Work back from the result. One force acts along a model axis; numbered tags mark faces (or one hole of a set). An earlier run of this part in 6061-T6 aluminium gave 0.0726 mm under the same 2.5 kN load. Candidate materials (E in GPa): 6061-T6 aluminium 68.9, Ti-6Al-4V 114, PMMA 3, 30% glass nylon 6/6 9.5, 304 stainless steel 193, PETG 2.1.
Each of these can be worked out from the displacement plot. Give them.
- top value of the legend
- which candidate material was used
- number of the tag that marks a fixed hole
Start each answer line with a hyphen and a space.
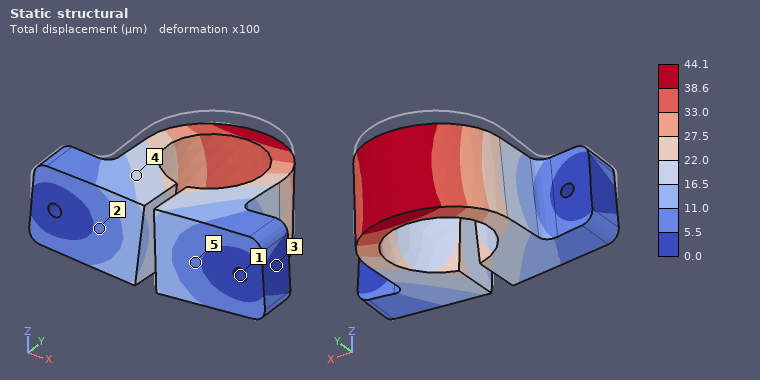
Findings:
- 44.1 µm
- Ti-6Al-4V
- 1
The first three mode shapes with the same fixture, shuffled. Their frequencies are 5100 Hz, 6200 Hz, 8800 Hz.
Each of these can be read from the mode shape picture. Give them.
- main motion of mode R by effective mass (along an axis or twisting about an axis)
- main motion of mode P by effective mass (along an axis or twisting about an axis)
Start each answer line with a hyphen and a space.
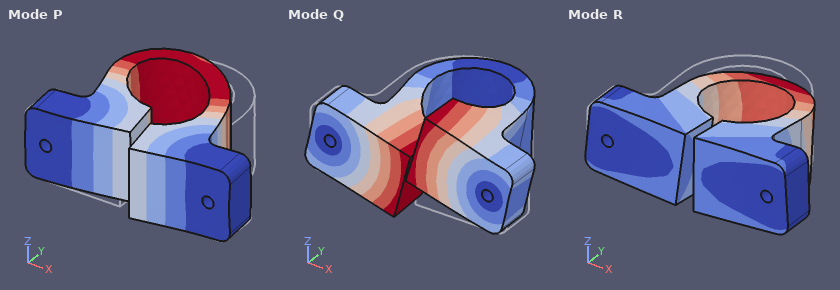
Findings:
- along Z
- along X
